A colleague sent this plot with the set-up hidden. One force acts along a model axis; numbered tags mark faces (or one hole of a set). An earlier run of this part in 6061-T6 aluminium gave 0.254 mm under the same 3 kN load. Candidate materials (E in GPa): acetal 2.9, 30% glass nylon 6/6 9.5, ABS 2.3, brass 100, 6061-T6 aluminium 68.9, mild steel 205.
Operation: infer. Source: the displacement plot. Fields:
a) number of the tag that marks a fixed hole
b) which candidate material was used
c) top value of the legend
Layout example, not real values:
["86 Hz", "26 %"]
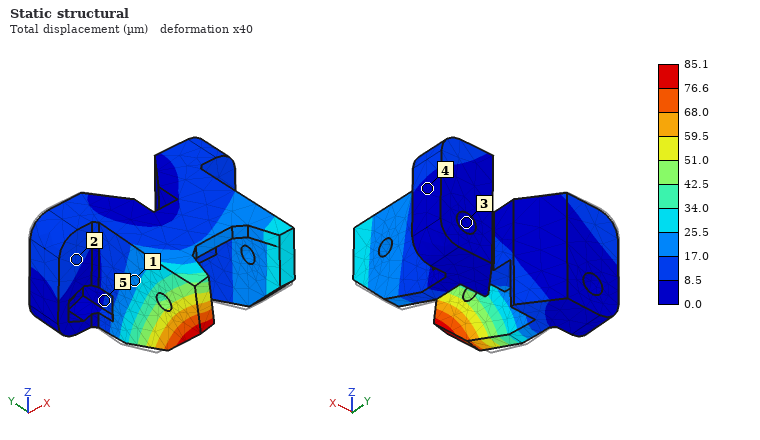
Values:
["3", "mild steel", "85.1 µm"]
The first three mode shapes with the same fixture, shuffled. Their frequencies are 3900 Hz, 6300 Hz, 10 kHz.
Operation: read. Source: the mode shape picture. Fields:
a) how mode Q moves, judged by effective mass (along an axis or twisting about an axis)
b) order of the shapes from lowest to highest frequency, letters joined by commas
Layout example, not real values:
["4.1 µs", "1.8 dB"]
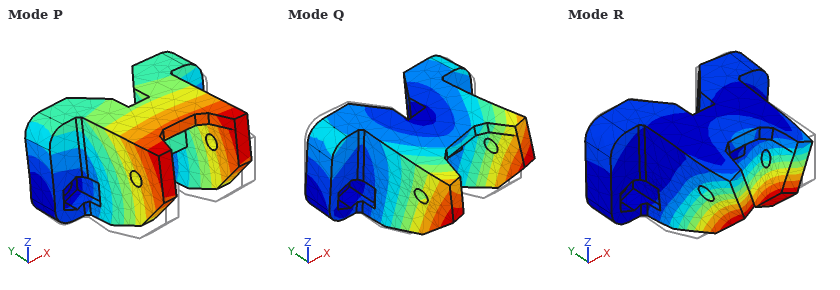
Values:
["along X", "P, Q, R"]
